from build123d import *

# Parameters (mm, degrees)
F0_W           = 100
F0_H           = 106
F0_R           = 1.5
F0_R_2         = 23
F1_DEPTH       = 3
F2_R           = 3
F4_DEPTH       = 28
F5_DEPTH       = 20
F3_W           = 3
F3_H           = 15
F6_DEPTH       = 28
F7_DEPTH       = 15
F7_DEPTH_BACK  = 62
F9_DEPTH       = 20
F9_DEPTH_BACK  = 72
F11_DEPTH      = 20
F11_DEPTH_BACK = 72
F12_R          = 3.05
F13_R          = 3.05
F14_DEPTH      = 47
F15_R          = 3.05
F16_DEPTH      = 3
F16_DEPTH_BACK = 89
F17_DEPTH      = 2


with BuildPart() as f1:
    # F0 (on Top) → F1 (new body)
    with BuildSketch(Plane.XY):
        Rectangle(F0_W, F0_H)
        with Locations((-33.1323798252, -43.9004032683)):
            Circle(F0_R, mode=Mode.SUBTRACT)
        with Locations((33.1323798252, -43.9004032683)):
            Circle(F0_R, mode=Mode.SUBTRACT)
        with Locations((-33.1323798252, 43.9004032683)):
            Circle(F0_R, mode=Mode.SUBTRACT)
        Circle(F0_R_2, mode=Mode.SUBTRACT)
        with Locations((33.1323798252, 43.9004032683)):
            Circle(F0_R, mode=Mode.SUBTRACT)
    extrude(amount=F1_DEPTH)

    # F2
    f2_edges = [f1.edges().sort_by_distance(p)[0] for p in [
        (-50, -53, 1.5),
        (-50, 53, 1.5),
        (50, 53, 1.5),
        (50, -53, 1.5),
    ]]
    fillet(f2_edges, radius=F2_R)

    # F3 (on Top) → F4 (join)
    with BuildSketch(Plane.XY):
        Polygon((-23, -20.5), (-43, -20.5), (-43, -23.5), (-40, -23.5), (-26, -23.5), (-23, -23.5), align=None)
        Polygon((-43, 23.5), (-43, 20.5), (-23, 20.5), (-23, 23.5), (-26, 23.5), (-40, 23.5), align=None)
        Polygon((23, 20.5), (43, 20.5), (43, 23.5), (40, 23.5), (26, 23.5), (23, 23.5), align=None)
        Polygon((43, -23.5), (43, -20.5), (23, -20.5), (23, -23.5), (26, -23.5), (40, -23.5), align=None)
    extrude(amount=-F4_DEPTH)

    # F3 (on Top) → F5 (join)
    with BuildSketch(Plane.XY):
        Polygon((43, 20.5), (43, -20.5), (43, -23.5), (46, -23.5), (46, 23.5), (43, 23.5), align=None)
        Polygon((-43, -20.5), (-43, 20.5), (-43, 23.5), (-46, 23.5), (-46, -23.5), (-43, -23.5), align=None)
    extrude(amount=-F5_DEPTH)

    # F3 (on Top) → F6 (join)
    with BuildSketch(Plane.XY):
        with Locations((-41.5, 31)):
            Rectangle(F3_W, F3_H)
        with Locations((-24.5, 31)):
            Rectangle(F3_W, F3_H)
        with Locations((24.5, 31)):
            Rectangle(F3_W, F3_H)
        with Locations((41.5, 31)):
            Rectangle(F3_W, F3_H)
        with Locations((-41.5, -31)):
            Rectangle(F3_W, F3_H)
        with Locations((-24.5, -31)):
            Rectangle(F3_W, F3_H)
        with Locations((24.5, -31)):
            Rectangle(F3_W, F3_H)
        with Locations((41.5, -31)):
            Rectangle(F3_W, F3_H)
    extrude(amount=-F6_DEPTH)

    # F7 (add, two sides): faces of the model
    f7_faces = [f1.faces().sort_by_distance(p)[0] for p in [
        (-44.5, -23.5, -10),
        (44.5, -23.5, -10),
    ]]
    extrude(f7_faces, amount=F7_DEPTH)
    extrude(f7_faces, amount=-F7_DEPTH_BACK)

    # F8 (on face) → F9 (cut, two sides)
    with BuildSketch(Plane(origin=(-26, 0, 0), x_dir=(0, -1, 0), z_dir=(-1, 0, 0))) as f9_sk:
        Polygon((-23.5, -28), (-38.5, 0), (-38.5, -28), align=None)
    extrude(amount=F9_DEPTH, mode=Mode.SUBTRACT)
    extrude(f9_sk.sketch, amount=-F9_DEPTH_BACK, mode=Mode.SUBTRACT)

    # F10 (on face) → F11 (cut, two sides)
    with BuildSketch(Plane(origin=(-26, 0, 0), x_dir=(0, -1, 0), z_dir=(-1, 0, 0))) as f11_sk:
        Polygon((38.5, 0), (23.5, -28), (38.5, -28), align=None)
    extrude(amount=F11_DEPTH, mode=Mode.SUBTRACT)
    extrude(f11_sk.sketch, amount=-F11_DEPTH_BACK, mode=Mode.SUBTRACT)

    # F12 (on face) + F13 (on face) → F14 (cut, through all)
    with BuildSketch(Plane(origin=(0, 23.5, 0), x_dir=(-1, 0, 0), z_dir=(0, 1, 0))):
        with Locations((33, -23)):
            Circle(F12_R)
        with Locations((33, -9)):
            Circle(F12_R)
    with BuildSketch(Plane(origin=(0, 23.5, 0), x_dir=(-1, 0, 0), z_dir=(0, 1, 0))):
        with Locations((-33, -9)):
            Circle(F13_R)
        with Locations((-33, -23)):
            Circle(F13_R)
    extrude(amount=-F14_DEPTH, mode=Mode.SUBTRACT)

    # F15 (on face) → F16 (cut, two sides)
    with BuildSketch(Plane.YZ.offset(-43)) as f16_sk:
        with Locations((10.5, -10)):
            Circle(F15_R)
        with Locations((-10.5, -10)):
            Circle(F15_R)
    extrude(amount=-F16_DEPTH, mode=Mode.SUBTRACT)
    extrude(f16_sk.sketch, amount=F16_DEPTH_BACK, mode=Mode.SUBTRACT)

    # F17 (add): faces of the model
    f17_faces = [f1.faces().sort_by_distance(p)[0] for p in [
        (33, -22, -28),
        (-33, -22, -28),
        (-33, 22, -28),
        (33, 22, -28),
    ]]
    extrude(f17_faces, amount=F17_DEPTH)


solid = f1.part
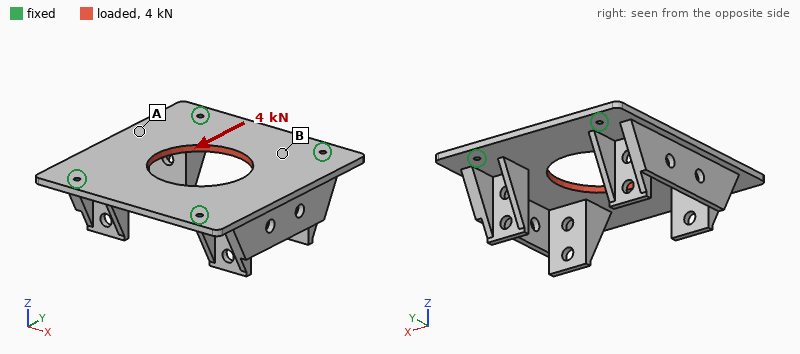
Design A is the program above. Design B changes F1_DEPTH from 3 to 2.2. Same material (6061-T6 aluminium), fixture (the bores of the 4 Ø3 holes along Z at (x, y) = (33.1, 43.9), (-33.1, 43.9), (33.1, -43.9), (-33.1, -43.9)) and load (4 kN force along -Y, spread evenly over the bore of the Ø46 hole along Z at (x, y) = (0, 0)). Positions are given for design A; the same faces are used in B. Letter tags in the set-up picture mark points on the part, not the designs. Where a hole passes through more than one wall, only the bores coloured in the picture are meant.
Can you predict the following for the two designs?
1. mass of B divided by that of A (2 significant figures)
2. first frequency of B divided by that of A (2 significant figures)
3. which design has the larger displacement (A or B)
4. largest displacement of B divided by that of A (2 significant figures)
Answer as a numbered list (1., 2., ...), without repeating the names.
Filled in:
1. 0.84
2. 0.74
3. B
4. 1.4
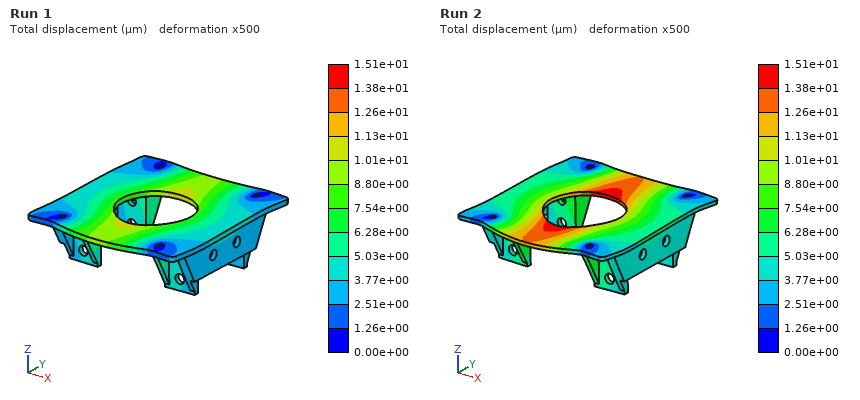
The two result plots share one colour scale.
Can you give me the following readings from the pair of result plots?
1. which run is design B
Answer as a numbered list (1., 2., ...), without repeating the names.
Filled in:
1. Run 2
